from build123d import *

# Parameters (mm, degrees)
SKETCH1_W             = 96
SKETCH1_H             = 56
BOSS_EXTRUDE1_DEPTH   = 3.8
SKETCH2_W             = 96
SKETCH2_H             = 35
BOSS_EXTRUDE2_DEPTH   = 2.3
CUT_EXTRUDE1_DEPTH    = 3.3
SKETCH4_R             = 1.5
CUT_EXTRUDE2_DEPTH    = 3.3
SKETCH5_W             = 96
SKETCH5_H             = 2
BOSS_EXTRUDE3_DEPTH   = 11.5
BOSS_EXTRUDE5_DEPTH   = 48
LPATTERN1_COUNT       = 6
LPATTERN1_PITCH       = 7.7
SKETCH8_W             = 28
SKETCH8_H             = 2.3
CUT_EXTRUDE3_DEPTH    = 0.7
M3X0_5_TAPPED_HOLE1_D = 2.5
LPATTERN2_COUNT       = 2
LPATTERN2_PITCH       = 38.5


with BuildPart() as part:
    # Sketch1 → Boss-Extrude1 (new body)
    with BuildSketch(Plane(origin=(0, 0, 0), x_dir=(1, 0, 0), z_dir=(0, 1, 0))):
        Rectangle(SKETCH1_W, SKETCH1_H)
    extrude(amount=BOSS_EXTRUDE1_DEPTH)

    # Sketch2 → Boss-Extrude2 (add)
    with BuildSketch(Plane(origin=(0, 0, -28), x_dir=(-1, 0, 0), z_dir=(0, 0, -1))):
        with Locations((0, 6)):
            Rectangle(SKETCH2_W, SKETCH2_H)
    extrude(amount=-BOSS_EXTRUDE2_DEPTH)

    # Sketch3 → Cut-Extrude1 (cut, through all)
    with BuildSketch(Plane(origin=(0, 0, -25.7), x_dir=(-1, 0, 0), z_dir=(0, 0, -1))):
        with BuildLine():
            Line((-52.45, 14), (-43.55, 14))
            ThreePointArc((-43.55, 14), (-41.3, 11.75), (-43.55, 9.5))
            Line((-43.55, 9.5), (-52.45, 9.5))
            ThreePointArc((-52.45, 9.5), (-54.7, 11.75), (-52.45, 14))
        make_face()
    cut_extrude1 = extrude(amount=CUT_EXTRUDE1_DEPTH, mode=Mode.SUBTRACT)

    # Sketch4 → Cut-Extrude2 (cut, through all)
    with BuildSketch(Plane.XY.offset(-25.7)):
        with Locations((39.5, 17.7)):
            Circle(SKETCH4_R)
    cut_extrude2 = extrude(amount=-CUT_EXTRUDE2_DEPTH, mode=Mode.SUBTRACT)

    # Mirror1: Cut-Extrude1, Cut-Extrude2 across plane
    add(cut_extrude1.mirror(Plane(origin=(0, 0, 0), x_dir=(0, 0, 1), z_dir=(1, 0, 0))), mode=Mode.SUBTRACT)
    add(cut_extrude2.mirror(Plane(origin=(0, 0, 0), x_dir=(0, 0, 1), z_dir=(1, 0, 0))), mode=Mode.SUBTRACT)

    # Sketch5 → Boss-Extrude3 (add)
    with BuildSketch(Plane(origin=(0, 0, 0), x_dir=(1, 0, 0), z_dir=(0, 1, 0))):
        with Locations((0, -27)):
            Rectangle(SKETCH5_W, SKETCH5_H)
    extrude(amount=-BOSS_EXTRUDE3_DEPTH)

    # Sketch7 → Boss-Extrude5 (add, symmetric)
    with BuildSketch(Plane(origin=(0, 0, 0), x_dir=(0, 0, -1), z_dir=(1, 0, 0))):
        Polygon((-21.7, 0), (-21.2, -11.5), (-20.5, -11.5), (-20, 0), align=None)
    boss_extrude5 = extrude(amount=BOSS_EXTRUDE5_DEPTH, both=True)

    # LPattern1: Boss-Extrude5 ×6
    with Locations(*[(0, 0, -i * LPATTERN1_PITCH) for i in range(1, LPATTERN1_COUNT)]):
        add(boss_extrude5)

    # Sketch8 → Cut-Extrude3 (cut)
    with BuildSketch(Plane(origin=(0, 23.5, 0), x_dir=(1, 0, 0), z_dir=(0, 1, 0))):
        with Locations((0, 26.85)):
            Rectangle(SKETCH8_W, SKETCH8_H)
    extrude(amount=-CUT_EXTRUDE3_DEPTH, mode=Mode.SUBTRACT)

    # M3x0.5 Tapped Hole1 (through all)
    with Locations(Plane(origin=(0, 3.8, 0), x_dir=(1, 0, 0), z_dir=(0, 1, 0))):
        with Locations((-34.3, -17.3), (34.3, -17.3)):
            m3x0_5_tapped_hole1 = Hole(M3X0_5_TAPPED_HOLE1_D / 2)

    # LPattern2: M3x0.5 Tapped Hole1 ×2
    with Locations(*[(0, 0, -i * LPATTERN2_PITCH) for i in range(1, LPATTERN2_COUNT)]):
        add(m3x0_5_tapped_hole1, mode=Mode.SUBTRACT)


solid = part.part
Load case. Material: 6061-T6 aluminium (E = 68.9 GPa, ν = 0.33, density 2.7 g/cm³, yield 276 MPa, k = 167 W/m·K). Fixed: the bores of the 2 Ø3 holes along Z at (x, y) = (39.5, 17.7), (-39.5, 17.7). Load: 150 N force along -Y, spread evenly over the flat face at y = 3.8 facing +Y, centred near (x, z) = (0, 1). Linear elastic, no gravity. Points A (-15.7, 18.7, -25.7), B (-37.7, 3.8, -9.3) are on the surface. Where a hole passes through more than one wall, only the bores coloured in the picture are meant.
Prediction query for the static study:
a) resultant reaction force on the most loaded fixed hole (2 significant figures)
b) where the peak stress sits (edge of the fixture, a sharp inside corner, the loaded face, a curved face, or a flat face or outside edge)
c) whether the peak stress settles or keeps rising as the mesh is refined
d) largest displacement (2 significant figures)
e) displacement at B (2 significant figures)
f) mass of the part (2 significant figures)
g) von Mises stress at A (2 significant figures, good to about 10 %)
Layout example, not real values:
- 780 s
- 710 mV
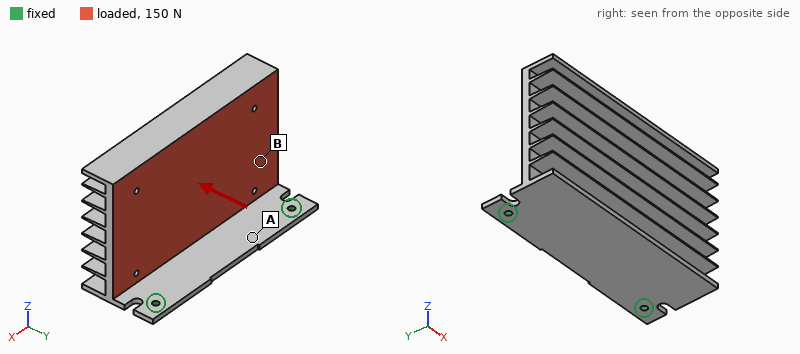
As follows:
- 85 N
- edge of the fixture
- keeps rising
- 1.3 mm
- 0.40 mm
- 100 g
- 36 MPa
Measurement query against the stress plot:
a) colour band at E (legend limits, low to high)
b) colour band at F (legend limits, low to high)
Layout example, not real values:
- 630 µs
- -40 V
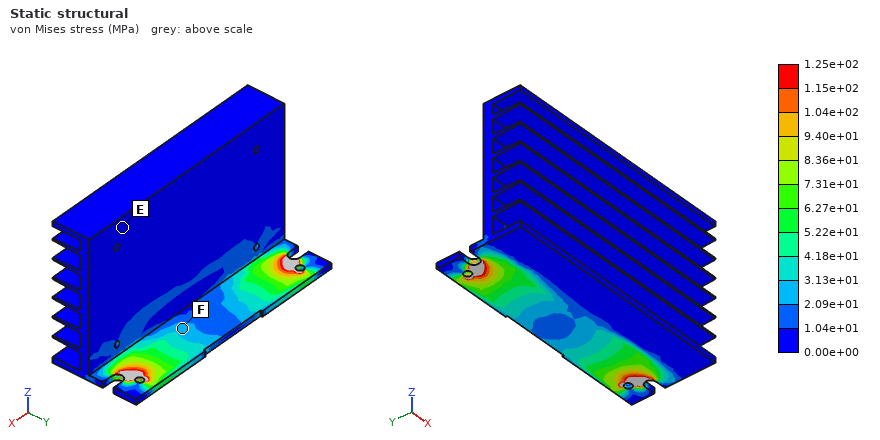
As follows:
- 0.00e+00 to 1.04e+01 MPa
- 2.09e+01 to 3.13e+01 MPa
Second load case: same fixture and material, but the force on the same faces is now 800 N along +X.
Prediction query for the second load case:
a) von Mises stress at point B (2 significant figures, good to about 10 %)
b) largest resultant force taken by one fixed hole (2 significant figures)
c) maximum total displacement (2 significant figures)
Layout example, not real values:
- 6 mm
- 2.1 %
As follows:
- 21 MPa
- 520 N
- 0.30 mm
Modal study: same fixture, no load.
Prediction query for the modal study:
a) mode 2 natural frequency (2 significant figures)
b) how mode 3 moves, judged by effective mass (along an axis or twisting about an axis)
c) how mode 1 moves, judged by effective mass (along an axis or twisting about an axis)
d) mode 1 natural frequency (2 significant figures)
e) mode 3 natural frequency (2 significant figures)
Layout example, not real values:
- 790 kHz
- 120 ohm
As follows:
- 880 Hz
- along X
- along Y
- 210 Hz
- 1300 Hz
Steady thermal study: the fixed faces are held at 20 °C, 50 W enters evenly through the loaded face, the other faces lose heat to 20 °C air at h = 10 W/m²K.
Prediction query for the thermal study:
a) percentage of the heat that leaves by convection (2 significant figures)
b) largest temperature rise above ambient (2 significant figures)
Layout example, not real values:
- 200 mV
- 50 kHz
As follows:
- 28 %
- 59 K
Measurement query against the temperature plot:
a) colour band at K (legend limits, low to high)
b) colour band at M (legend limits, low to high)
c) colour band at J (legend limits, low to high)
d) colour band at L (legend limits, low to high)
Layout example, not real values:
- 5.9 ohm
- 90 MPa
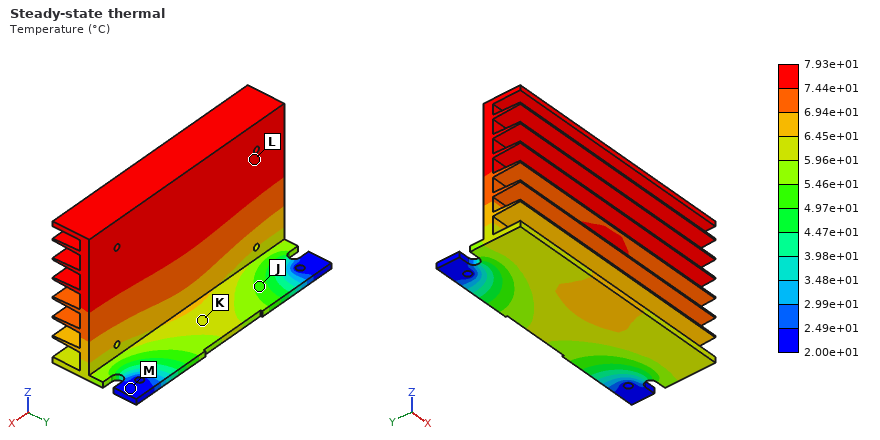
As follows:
- 5.96e+01 to 6.45e+01 °C
- 2.00e+01 to 2.49e+01 °C
- 4.97e+01 to 5.46e+01 °C
- 7.44e+01 to 7.93e+01 °C
